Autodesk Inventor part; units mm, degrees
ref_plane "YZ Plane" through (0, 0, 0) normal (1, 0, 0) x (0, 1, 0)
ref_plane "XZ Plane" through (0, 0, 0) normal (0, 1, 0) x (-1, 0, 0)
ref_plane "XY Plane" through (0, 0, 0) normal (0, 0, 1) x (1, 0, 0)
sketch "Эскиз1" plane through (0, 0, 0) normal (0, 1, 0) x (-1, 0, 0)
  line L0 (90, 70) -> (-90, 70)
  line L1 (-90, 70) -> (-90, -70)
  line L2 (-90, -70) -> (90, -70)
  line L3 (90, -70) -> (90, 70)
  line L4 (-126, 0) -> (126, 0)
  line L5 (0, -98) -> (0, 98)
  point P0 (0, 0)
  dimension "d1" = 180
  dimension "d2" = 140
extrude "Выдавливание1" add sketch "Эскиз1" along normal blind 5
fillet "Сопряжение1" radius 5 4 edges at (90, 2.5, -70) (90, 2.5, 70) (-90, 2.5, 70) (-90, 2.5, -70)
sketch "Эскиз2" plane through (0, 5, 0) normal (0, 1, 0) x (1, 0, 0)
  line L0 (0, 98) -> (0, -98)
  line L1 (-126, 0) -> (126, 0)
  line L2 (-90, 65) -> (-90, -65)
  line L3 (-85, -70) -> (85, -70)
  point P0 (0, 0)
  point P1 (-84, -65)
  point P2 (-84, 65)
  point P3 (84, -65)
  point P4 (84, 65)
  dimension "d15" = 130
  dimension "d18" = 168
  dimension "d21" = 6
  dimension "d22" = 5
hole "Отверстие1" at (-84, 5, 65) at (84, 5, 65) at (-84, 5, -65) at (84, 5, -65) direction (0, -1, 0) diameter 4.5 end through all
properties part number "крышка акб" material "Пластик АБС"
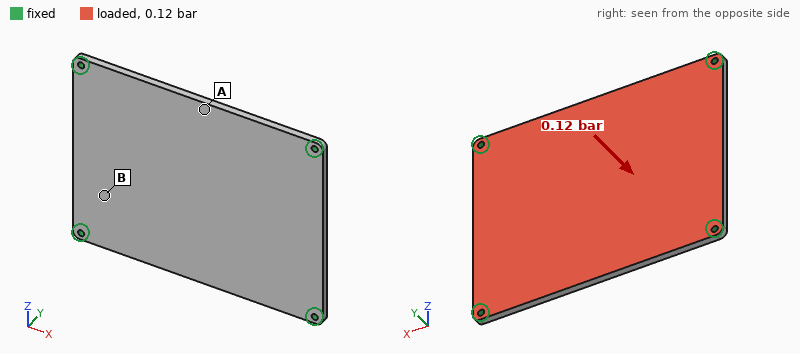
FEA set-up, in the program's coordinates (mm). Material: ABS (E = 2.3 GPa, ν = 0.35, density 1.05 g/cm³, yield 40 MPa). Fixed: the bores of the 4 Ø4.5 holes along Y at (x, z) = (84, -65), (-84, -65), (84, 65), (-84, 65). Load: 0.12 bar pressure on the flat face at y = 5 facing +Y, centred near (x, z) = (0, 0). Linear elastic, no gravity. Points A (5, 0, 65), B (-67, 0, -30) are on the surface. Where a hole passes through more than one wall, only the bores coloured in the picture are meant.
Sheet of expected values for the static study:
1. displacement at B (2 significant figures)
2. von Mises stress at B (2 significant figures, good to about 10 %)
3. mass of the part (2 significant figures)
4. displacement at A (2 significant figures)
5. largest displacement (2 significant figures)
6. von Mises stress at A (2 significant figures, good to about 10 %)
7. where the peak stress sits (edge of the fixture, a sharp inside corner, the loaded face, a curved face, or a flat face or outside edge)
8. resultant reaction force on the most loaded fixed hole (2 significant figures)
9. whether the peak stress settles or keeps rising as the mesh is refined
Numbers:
0.91 mm
2.1 MPa
130 g
1.9 mm
2.3 mm
5.5 MPa
edge of the fixture
75 N
keeps rising
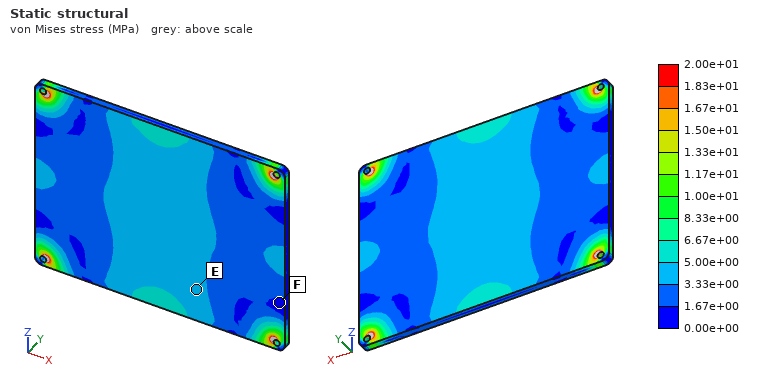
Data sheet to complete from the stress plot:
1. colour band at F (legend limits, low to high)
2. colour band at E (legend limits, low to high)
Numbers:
0.00e+00 to 1.67e+00 MPa
3.33e+00 to 5.00e+00 MPa
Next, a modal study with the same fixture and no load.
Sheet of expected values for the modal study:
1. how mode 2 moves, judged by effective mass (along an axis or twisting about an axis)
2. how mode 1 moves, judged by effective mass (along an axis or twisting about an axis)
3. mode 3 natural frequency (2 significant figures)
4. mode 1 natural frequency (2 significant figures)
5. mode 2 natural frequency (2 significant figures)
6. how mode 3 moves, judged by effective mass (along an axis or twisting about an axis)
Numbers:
twisting about X
along Y
410 Hz
180 Hz
320 Hz
twisting about Z
